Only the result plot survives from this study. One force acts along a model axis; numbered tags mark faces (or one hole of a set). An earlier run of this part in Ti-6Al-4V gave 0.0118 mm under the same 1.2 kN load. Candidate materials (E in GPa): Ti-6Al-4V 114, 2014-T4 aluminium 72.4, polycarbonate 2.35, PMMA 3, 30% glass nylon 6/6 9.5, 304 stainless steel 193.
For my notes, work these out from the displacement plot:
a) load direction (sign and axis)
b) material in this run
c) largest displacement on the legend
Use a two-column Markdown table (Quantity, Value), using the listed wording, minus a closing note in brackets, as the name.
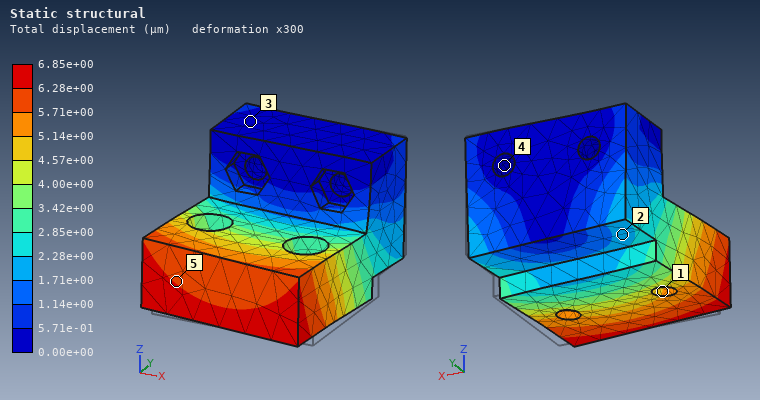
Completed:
| Quantity | Value |
|---|---|
| load direction | -X |
| material in this run | 304 stainless steel |
| largest displacement on the legend | 6.85e+00 µm |
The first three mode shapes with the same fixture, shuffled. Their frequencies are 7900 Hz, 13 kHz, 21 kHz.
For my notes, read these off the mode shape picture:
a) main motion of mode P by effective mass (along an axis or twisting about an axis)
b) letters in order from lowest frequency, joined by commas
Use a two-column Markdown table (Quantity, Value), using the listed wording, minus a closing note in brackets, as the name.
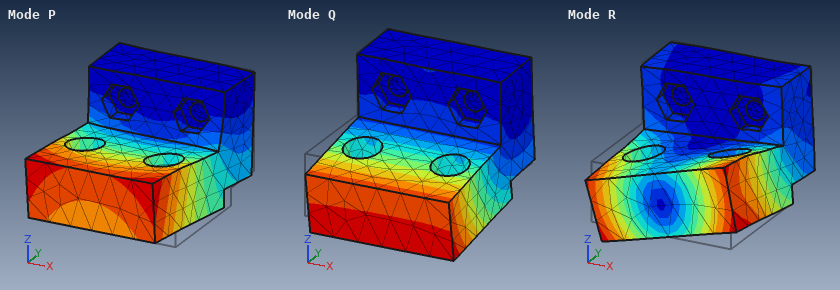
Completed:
| Quantity | Value |
|---|---|
| main motion of mode P by effective mass | along X |
| letters in order from lowest frequency, joined by commas | Q, P, R |
